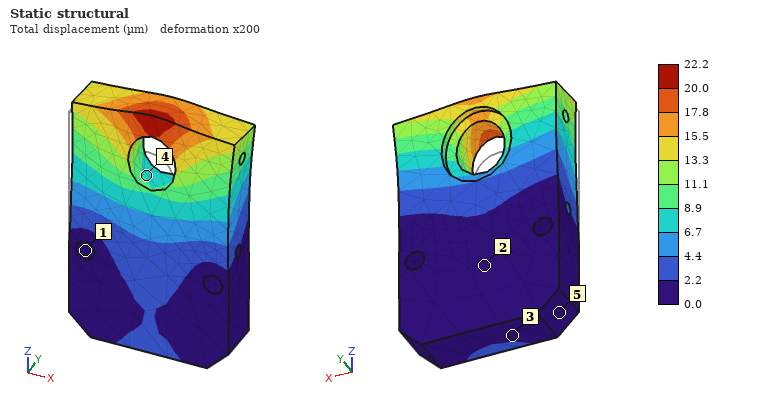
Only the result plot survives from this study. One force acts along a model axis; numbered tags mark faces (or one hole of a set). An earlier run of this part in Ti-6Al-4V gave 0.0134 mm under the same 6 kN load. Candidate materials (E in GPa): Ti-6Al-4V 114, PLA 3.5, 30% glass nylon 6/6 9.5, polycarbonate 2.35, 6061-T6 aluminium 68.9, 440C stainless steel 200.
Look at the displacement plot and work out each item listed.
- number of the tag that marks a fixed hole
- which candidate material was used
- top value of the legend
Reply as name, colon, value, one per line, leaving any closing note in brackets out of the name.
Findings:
number of the tag that marks a fixed hole: 1
which candidate material was used: 6061-T6 aluminium
top value of the legend: 22.2 µm
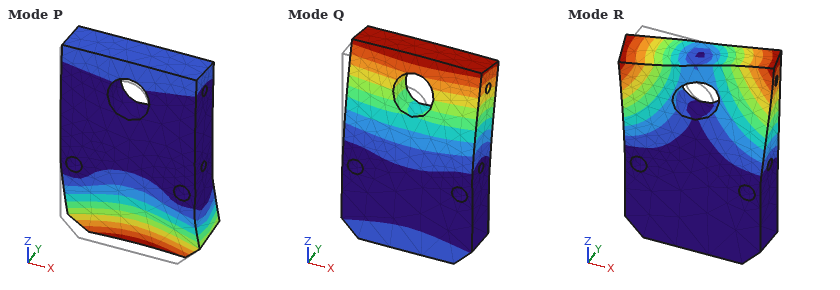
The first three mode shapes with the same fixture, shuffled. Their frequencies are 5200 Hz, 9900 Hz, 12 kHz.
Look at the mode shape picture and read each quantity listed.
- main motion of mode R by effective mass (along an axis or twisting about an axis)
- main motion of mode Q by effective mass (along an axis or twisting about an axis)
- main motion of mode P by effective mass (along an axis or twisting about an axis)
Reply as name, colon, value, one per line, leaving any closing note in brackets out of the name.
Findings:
main motion of mode R by effective mass: twisting about Z
main motion of mode Q by effective mass: along Y
main motion of mode P by effective mass: along Y
